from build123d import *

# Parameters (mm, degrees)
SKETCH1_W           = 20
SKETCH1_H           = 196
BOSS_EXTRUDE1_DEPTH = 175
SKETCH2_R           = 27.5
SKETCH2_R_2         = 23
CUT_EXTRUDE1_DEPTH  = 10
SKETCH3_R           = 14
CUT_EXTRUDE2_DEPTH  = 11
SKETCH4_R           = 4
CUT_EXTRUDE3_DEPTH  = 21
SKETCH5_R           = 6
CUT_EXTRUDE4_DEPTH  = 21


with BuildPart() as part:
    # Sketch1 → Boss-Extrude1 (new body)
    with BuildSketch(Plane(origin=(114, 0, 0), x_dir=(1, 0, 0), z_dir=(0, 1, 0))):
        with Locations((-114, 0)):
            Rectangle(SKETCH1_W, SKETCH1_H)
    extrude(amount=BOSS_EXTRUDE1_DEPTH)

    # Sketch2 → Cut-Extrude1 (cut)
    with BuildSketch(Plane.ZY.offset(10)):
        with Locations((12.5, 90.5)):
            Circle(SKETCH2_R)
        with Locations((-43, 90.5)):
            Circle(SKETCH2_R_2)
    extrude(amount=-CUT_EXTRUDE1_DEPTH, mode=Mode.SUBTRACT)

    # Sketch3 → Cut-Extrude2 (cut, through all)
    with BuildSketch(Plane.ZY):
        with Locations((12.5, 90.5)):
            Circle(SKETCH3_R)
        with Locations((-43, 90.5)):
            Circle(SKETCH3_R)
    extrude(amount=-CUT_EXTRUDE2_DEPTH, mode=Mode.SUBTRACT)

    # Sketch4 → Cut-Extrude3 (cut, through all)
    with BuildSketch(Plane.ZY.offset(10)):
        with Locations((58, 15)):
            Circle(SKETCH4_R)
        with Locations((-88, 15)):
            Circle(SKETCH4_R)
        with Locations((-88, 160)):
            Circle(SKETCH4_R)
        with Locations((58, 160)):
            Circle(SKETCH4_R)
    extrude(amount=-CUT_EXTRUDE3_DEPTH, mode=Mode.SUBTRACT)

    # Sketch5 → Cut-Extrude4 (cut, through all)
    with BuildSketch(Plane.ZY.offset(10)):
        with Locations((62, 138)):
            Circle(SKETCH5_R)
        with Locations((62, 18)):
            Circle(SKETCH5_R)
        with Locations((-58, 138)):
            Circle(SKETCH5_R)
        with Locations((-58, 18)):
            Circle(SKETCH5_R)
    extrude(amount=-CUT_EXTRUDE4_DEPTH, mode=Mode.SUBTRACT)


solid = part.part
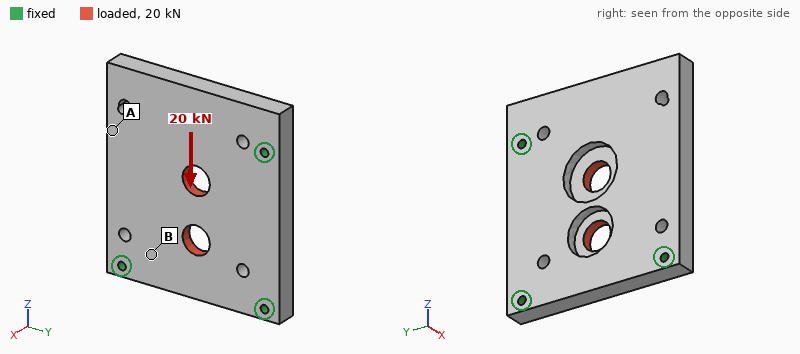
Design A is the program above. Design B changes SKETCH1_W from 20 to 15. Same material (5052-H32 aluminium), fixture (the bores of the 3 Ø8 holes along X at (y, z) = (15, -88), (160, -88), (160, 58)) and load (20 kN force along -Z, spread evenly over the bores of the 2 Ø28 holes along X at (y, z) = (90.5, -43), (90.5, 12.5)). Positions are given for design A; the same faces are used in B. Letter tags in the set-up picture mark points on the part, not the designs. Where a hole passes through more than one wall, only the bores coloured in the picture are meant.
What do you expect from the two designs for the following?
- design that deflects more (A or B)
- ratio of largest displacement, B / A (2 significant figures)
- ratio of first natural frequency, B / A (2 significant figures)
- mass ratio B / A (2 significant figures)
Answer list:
B
1.6
0.78
0.75
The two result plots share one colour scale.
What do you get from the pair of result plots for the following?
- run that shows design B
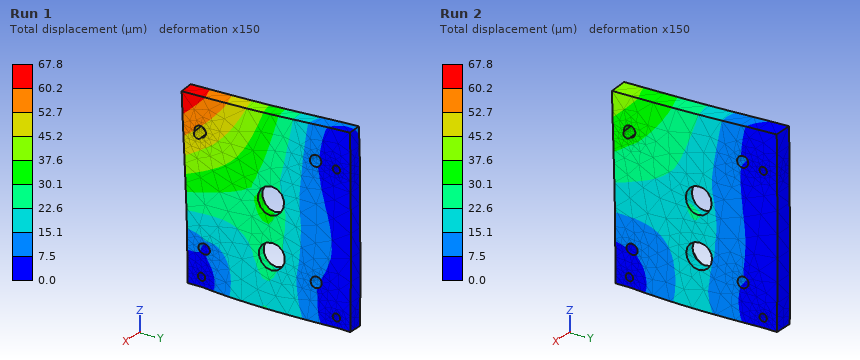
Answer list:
Run 1
